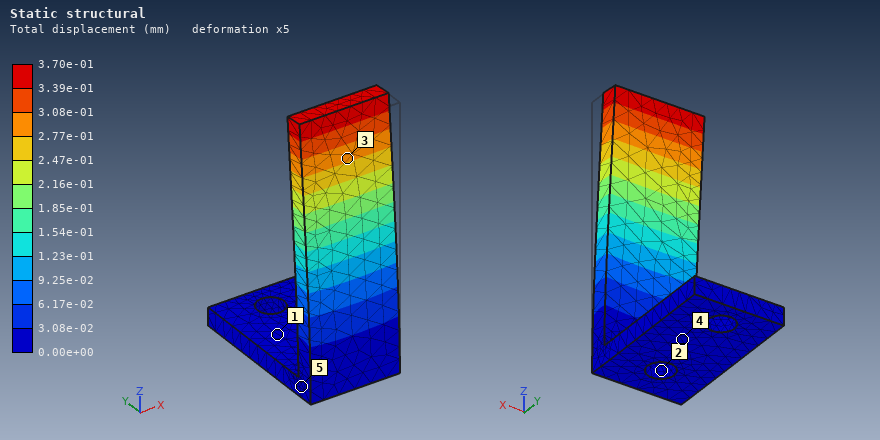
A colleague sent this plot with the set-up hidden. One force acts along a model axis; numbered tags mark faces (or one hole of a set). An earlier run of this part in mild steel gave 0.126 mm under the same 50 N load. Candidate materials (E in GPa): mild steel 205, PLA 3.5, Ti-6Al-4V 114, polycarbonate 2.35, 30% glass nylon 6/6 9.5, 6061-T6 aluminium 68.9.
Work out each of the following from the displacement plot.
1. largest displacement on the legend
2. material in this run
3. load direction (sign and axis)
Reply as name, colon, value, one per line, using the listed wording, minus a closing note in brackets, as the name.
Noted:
largest displacement on the legend: 3.70e-01 mm
material in this run: 6061-T6 aluminium
load direction: +Y
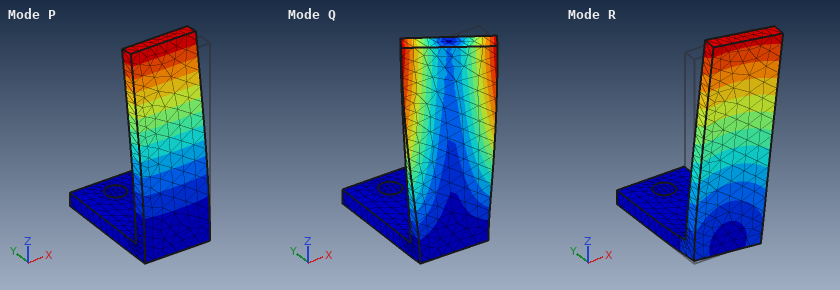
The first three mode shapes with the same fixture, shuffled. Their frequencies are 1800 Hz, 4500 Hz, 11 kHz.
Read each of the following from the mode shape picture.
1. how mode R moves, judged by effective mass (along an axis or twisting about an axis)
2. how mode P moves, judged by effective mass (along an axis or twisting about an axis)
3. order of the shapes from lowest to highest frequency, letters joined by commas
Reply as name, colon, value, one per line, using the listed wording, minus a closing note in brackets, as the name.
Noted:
how mode R moves, judged by effective mass: along X
how mode P moves, judged by effective mass: along Y
order of the shapes from lowest to highest frequency, letters joined by commas: P, R, Q
